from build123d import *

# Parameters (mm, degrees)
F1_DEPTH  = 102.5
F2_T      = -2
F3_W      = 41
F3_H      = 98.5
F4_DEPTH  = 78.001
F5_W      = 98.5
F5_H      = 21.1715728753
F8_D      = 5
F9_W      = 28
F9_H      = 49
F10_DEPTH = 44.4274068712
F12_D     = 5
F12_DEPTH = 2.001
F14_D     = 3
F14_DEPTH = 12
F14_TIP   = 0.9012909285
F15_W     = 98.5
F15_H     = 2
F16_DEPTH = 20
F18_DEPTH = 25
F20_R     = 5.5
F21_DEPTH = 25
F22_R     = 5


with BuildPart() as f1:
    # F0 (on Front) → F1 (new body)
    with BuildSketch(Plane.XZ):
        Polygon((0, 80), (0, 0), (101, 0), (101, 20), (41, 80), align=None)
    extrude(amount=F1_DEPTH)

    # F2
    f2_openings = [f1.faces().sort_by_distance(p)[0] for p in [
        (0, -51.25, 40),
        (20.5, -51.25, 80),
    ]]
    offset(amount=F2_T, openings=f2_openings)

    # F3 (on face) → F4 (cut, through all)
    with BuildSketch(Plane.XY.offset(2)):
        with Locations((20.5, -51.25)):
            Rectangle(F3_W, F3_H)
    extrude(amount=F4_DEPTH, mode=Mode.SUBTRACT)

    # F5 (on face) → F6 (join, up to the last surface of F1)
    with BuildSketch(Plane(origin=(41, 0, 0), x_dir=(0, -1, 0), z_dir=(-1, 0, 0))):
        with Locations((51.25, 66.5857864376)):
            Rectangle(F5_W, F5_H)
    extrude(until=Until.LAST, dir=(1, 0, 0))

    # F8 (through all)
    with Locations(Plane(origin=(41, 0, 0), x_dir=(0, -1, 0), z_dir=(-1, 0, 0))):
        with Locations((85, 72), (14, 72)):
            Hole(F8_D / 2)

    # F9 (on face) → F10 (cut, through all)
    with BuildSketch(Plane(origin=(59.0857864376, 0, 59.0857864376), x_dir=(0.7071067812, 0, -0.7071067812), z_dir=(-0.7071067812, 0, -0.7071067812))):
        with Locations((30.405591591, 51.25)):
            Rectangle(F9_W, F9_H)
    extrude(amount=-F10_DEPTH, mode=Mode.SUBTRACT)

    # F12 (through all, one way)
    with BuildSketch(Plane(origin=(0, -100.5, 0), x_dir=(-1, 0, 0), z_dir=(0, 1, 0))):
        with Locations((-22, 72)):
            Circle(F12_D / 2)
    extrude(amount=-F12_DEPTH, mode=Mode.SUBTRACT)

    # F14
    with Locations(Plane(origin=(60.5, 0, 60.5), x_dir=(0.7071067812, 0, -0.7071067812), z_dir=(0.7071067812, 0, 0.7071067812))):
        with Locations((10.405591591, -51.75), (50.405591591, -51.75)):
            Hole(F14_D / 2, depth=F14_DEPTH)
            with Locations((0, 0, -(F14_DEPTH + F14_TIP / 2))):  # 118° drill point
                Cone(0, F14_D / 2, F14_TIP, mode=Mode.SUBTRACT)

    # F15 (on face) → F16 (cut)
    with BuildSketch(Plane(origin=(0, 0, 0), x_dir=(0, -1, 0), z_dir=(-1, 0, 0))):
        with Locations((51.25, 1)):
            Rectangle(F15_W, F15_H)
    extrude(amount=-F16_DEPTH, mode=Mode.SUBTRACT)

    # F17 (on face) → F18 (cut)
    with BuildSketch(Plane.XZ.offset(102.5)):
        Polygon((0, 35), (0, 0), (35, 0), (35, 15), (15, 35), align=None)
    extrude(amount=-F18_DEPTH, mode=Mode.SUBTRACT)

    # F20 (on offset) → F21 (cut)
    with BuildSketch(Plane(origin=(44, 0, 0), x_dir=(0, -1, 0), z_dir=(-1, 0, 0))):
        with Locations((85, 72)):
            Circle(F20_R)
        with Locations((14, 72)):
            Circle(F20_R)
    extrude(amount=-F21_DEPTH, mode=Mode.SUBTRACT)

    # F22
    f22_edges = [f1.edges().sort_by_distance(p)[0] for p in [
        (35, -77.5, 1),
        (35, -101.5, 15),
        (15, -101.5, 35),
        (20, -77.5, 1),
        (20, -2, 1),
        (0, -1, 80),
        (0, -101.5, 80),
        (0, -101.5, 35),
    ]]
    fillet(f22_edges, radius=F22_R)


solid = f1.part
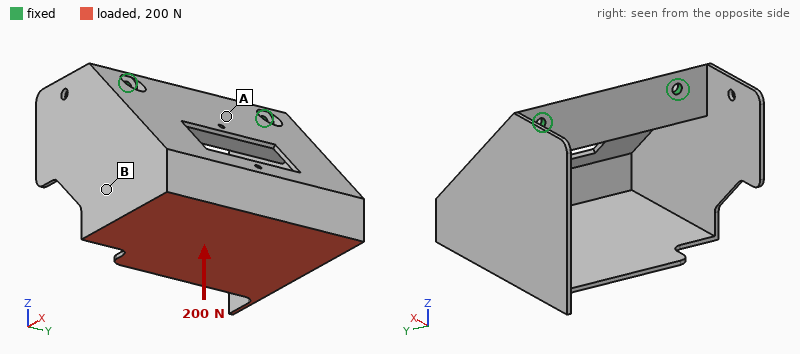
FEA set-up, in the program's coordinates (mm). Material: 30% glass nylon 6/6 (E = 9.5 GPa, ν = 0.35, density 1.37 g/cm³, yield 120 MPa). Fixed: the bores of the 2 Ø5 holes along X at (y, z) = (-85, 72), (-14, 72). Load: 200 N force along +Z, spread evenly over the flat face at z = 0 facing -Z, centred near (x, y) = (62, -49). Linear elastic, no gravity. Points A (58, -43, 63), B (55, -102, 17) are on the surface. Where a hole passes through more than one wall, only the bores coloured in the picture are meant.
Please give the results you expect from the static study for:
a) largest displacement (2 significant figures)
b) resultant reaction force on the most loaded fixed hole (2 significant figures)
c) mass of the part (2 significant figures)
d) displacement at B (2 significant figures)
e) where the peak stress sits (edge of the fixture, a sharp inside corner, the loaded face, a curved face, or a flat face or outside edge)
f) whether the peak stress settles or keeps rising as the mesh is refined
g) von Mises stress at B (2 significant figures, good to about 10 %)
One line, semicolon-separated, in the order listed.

2.0 mm; 100 N; 100 g; 0.51 mm; edge of the fixture; keeps rising; 8.1 MPa
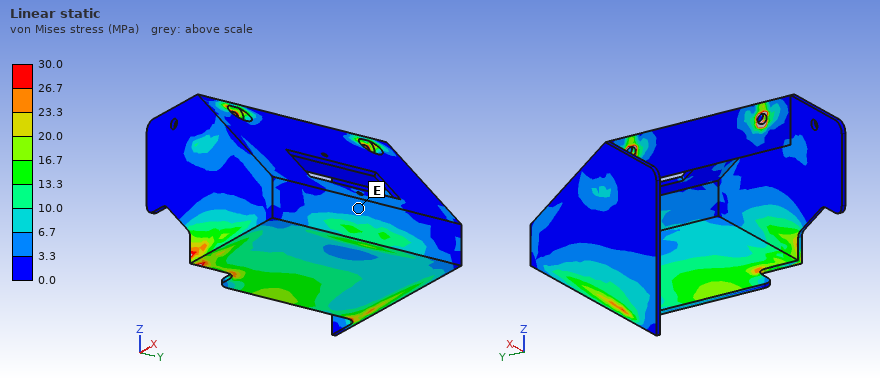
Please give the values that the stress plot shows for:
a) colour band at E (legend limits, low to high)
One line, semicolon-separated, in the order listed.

3.3 to 6.7 MPa
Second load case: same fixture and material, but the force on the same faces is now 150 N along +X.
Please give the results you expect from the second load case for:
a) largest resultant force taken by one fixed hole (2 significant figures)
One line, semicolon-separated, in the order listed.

130 N
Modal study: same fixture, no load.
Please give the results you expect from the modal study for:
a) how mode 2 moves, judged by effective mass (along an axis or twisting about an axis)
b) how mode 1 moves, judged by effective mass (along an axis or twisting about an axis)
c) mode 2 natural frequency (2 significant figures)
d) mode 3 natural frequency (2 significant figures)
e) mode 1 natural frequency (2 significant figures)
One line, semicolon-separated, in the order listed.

along Y; along X; 320 Hz; 440 Hz; 220 Hz
